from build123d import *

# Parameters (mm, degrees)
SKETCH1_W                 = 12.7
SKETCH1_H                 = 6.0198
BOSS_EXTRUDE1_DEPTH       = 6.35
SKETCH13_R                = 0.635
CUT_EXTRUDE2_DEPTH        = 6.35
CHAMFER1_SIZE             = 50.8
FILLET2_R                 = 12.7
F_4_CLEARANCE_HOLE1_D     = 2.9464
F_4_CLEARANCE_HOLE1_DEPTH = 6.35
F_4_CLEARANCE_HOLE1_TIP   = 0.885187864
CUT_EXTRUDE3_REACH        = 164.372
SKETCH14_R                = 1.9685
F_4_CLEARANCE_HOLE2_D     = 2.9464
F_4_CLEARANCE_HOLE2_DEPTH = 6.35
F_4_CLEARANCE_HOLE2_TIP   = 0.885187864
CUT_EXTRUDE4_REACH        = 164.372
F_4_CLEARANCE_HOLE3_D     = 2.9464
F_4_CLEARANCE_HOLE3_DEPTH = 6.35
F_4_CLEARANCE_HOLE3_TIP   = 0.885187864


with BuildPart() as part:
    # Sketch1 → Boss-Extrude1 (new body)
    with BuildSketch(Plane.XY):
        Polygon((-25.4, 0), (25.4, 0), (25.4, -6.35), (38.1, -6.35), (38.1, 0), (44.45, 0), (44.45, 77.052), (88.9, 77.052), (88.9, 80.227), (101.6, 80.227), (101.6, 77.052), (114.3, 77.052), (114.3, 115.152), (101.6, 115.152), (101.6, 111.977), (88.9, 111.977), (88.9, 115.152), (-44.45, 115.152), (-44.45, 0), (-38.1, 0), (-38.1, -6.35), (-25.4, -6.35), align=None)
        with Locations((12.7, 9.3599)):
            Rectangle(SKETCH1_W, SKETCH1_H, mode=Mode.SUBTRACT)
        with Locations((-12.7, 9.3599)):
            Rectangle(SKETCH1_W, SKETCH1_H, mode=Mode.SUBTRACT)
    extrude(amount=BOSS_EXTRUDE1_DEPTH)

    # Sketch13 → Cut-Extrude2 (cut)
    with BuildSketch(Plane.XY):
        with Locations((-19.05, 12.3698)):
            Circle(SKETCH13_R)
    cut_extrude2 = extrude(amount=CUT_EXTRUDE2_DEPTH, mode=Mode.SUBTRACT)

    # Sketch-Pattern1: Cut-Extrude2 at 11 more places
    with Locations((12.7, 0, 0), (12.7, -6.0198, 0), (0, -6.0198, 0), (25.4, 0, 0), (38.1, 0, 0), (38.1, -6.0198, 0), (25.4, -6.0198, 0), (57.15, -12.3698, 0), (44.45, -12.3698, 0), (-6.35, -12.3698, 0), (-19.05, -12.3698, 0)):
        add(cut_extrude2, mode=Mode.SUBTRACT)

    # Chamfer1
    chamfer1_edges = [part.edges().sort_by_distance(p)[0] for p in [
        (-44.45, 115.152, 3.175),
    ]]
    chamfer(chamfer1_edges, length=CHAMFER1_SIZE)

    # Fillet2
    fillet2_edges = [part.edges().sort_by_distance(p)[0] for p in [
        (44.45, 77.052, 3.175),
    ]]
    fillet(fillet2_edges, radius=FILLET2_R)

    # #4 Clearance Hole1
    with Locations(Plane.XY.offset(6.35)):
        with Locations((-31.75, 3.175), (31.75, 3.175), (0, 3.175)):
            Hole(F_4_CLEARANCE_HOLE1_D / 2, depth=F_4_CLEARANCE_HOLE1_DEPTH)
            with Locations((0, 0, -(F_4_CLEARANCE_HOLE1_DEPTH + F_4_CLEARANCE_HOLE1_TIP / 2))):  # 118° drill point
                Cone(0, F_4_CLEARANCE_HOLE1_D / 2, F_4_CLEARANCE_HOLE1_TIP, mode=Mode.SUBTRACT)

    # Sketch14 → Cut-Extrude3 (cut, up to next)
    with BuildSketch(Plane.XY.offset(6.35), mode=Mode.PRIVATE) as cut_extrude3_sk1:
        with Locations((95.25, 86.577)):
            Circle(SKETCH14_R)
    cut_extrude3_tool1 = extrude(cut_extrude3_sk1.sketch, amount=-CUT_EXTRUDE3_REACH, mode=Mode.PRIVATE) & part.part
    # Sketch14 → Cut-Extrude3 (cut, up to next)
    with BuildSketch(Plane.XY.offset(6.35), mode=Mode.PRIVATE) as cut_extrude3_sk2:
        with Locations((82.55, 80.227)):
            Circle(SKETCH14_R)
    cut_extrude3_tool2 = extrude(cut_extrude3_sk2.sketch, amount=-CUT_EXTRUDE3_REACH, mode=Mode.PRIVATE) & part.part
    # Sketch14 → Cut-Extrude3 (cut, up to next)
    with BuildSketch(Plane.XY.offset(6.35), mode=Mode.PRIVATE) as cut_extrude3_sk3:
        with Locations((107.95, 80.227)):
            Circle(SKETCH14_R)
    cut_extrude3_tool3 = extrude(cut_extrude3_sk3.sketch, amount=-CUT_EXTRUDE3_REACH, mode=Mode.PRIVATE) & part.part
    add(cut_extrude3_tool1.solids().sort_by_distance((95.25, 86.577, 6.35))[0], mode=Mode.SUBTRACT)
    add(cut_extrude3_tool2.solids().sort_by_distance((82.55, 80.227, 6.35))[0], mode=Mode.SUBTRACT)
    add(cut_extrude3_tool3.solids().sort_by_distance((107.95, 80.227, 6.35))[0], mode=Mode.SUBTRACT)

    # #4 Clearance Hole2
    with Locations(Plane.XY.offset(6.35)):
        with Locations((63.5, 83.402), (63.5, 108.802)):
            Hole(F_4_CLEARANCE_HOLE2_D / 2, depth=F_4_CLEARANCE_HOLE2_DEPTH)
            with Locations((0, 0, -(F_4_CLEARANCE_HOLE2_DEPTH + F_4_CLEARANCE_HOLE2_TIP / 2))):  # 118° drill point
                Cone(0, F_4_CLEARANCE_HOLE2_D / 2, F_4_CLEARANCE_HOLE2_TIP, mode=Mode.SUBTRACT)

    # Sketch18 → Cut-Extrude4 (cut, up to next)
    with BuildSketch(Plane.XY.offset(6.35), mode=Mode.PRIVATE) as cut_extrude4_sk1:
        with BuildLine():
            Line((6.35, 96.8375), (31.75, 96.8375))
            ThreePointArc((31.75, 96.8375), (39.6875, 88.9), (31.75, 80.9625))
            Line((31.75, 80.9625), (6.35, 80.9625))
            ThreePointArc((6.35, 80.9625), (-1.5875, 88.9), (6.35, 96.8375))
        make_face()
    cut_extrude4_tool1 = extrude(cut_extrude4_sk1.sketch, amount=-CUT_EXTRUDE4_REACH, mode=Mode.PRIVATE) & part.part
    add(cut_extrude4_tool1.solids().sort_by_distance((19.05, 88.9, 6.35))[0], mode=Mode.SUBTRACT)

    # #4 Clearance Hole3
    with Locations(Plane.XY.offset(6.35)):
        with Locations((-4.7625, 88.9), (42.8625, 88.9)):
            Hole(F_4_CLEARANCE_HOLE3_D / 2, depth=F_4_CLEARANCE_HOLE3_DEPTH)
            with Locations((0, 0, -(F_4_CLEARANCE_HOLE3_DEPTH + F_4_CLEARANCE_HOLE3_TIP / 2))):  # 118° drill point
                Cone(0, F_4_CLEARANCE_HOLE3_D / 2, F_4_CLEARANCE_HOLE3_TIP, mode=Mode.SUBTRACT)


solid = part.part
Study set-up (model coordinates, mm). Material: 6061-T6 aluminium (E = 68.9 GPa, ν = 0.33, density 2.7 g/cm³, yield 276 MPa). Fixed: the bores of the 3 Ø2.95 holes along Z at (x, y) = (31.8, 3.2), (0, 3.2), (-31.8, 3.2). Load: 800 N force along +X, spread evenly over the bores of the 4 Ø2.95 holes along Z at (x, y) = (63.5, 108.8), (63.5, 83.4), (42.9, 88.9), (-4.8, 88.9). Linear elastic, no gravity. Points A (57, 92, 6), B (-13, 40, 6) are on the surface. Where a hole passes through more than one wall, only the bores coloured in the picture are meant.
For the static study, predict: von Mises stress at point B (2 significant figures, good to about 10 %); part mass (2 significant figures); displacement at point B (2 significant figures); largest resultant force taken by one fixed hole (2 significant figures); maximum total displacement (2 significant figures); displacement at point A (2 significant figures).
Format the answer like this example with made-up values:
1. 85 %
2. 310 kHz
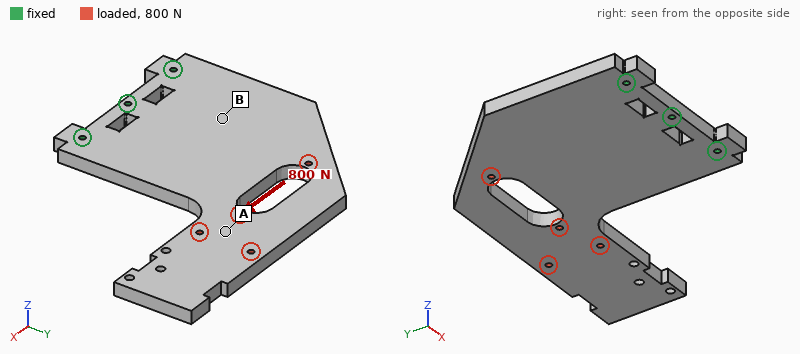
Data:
1. 4.1 MPa
2. 190 g
3. 7.2 µm
4. 1.1 kN
5. 44 µm
6. 27 µm
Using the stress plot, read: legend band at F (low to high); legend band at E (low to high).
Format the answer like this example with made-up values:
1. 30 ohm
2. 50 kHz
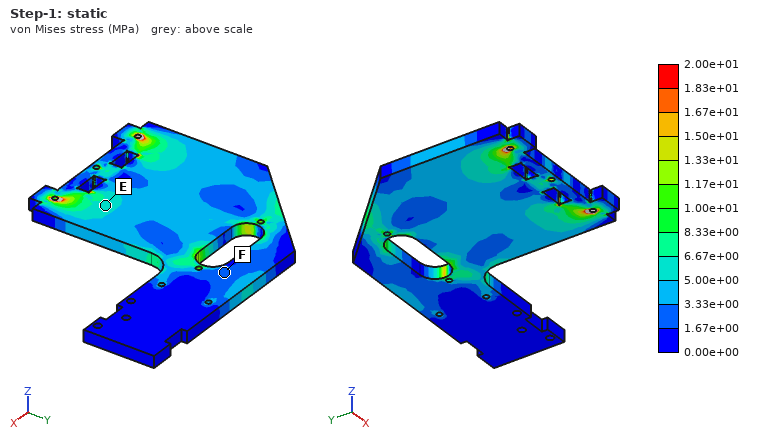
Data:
1. 1.67e+00 to 3.33e+00 MPa
2. 5.00e+00 to 6.67e+00 MPa
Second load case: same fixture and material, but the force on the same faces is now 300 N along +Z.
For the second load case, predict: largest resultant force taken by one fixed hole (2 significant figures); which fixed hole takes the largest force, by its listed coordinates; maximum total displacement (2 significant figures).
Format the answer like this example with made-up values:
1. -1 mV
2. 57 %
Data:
1. 280 N
2. (31.8, 3.2)
3. 1.7 mm
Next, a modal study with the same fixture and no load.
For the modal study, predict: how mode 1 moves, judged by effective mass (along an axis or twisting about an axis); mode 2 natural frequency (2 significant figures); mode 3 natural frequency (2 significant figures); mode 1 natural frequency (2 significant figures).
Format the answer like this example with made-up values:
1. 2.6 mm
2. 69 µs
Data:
1. along Z
2. 640 Hz
3. 1700 Hz
4. 270 Hz
